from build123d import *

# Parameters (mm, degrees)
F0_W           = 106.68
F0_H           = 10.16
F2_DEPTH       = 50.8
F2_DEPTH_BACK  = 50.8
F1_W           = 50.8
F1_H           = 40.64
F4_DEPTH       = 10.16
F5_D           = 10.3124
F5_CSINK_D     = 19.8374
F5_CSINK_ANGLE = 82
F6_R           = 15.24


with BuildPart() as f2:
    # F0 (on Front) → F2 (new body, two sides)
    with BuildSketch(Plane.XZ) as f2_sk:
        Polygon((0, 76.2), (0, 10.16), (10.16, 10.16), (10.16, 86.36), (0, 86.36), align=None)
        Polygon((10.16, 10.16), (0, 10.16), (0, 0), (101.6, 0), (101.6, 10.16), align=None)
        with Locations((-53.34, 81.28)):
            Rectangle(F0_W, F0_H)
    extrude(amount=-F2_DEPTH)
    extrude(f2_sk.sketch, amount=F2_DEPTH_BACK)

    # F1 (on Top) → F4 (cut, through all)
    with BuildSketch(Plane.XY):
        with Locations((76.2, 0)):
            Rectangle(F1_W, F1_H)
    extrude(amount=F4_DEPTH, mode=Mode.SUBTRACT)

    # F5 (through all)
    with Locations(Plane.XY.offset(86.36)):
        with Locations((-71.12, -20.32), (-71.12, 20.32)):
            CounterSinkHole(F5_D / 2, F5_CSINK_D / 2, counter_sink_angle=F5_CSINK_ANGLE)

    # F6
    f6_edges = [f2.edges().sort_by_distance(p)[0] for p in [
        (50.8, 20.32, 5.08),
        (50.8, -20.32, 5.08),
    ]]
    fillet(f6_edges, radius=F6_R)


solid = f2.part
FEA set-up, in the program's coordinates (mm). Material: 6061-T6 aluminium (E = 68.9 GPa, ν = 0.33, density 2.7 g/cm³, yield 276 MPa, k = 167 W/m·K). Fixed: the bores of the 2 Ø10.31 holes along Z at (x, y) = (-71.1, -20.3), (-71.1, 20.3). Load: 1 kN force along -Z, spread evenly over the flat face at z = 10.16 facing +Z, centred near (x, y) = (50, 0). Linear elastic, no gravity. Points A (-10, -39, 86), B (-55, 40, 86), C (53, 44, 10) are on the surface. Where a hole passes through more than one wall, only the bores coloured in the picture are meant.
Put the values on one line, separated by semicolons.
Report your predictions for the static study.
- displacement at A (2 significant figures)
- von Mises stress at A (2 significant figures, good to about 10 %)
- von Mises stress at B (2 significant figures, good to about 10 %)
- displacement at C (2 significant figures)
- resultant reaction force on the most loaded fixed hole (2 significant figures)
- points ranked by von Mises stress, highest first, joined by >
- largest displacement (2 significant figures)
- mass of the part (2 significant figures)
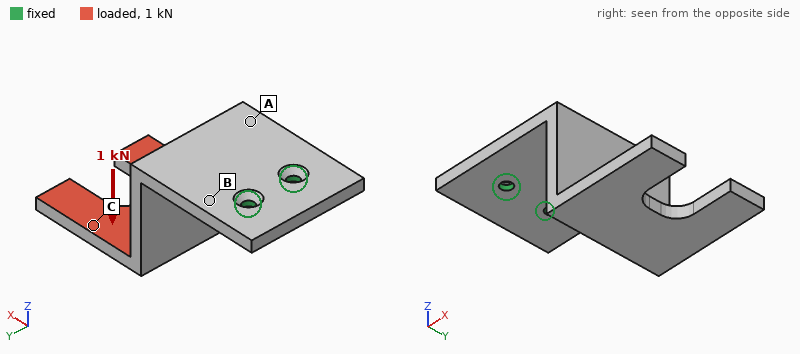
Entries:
0.46 mm; 32 MPa; 58 MPa; 1.8 mm; 660 N; B > A > C; 2.8 mm; 730 g
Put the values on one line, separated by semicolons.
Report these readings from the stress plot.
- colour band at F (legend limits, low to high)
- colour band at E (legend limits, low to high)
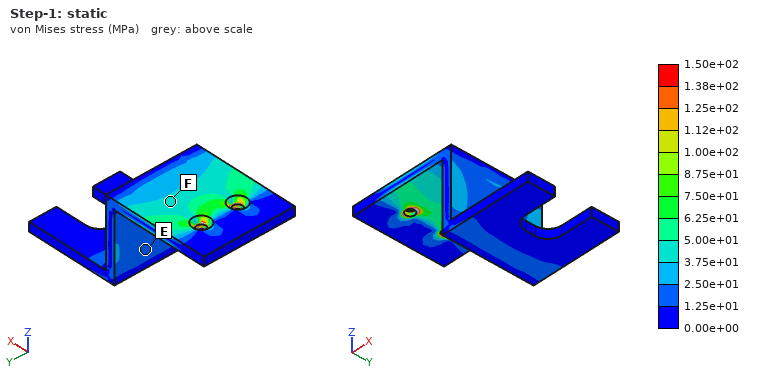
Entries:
3.75e+01 to 5.00e+01 MPa; 1.25e+01 to 2.50e+01 MPa
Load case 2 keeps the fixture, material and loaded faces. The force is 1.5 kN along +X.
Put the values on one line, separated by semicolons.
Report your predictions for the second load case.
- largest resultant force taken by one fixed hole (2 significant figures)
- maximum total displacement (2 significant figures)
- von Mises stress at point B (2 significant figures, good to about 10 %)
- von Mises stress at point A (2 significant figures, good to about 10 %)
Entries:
1.0 kN; 2.9 mm; 58 MPa; 55 MPa
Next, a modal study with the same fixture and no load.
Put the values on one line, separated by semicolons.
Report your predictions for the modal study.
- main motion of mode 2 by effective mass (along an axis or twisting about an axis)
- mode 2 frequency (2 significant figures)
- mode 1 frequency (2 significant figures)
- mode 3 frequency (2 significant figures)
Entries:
along Y; 430 Hz; 200 Hz; 780 Hz
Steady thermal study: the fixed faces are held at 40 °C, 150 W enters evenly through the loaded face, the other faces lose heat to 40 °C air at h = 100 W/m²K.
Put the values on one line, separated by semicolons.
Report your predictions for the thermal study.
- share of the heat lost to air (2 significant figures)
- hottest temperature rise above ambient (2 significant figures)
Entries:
82 %; 62 K
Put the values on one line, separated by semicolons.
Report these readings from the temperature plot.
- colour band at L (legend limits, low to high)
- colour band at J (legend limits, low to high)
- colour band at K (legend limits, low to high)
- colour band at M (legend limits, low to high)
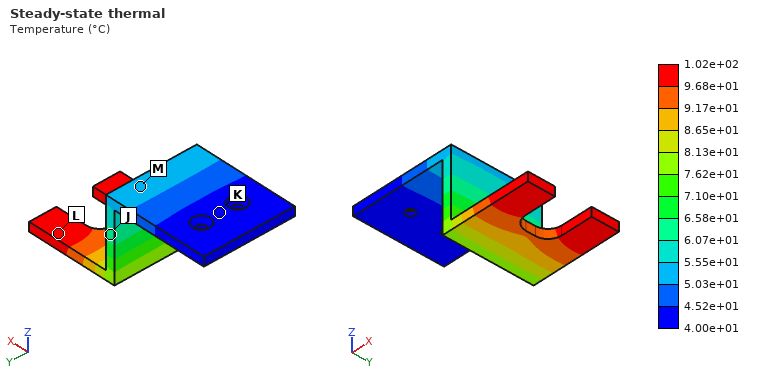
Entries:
9.68e+01 to 1.02e+02 °C; 6.07e+01 to 6.58e+01 °C; 4.00e+01 to 4.52e+01 °C; 5.03e+01 to 5.55e+01 °C
